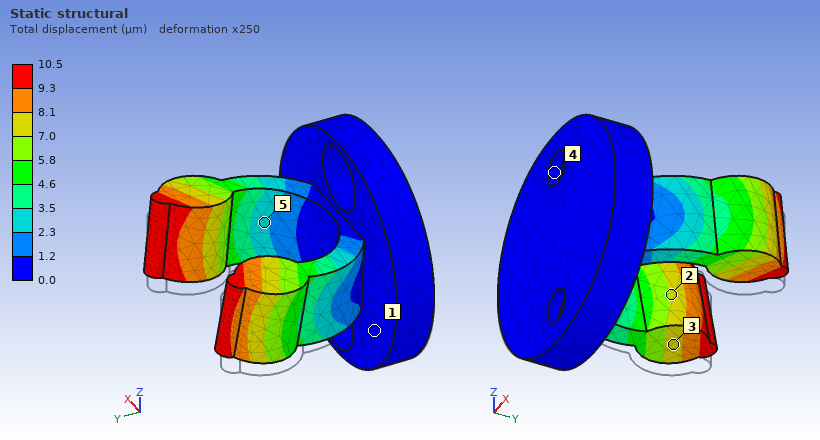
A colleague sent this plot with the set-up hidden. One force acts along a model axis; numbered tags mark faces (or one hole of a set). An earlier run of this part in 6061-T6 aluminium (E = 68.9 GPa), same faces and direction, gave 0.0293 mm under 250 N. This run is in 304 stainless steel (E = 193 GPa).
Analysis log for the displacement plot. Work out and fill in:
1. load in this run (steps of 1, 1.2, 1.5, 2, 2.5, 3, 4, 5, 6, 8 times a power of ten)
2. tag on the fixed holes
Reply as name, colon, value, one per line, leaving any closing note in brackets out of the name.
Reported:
load in this run: 250 N
tag on the fixed holes: 4
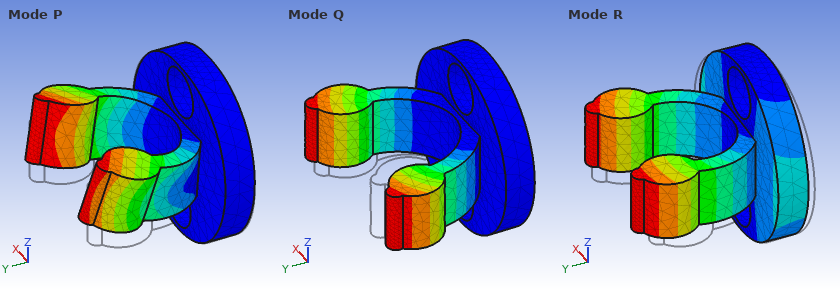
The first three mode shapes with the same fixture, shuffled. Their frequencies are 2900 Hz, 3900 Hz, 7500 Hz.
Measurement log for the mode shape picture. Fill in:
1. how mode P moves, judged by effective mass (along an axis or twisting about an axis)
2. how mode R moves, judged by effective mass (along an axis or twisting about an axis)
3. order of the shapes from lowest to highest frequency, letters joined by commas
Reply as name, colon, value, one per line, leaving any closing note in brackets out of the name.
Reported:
how mode P moves, judged by effective mass: along Z
how mode R moves, judged by effective mass: along X
order of the shapes from lowest to highest frequency, letters joined by commas: R, Q, P
